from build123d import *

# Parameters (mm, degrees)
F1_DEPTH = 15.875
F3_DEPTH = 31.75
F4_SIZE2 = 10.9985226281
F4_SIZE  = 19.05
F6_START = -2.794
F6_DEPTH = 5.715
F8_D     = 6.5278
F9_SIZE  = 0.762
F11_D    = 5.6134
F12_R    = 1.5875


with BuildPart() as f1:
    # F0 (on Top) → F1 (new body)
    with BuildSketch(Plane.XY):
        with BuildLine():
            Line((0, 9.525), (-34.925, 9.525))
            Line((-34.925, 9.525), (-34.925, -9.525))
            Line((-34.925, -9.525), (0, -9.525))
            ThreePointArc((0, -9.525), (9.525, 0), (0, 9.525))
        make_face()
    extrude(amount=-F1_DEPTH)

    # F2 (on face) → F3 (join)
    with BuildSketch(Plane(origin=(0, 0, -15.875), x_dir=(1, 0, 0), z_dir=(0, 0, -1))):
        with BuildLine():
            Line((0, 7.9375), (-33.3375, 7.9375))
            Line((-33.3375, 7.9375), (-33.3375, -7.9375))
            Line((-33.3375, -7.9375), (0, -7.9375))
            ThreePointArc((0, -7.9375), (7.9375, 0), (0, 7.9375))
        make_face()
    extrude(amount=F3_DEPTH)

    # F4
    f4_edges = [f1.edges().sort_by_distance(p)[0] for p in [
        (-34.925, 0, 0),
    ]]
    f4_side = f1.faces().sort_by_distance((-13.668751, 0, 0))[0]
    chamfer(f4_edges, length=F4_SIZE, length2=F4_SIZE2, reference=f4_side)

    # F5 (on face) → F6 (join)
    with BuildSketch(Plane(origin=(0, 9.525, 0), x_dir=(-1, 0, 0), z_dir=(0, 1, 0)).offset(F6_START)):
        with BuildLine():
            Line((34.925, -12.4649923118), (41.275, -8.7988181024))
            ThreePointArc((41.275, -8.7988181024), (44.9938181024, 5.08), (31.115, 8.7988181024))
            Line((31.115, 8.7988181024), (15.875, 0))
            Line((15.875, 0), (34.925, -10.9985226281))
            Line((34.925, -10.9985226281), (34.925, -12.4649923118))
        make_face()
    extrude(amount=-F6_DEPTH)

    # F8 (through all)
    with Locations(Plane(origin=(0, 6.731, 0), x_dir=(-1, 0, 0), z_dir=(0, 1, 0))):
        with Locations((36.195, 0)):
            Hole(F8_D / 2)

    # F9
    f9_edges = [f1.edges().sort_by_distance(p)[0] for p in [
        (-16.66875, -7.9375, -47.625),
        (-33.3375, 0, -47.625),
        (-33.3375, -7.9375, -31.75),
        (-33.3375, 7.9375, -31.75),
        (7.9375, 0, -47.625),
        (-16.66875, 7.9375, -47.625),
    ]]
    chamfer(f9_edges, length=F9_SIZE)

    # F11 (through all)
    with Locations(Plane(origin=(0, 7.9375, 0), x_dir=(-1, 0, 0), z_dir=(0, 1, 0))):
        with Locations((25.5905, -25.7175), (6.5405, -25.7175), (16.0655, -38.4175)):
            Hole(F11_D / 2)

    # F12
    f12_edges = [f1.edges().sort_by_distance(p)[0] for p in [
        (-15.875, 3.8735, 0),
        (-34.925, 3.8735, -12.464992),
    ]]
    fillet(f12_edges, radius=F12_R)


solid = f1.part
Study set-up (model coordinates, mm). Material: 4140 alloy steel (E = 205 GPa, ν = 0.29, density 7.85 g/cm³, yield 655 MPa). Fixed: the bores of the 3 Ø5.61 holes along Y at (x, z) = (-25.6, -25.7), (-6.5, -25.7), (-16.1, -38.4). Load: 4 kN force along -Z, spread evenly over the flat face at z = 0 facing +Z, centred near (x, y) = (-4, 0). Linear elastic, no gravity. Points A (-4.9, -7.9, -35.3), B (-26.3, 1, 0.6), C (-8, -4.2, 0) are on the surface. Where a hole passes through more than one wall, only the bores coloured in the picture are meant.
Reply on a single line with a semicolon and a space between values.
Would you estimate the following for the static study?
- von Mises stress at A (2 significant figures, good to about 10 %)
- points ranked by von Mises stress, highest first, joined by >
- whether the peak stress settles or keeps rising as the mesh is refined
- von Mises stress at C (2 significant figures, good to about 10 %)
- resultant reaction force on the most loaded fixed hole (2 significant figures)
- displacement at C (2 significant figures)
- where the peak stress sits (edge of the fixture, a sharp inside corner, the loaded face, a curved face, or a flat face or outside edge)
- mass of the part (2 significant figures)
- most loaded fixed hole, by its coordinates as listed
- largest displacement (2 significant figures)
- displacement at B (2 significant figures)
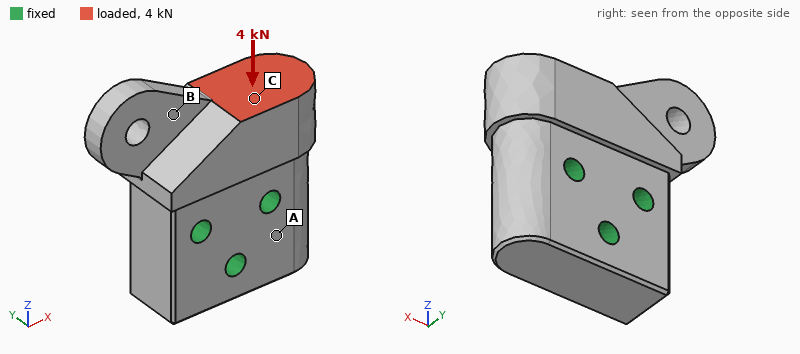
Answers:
4.7 MPa; C > A > B; keeps rising; 8.4 MPa; 3.7 kN; 1.7 µm; edge of the fixture; 250 g; (-6.5, -25.7); 2.6 µm; 1.0 µm
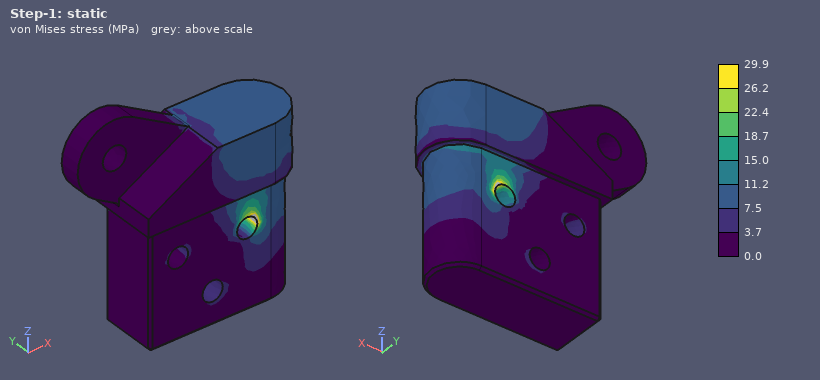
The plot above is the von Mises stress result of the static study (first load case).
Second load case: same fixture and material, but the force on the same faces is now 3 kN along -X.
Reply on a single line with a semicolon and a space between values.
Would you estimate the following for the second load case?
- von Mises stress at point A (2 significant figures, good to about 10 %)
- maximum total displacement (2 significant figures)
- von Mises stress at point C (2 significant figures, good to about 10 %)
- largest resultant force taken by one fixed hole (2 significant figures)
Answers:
5.8 MPa; 5.2 µm; 16 MPa; 3.4 kN
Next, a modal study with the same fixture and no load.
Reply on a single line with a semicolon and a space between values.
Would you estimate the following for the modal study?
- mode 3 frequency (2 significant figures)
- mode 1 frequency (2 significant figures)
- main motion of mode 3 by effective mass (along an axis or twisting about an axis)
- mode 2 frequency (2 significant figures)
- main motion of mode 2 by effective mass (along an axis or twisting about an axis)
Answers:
17 kHz; 9300 Hz; along X; 15 kHz; along Y
